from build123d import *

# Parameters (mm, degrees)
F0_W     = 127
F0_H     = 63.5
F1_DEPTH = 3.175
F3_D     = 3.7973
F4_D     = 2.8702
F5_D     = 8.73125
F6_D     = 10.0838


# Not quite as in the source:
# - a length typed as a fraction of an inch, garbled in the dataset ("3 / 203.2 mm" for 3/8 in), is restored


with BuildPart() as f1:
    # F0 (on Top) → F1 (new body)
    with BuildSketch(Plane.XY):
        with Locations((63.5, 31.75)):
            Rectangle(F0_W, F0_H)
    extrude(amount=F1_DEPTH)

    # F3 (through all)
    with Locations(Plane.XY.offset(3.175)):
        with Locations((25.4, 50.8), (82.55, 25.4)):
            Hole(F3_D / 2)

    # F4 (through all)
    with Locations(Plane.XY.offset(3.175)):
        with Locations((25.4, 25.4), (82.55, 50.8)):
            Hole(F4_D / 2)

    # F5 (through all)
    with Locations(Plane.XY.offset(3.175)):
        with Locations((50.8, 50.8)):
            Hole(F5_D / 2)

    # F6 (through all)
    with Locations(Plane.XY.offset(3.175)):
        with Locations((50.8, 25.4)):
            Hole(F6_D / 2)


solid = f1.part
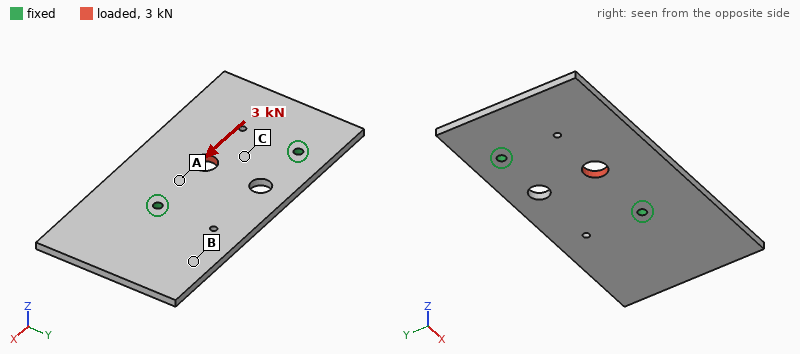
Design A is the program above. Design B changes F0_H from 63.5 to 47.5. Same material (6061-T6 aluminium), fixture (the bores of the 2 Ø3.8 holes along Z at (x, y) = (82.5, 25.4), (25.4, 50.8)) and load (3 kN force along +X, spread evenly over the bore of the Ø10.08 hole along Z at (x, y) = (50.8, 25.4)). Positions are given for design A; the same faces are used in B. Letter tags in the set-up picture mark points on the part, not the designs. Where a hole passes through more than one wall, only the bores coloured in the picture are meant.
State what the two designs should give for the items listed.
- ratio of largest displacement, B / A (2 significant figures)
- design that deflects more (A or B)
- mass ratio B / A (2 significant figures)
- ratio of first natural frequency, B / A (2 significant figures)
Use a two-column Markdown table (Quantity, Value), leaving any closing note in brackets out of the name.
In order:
| Quantity | Value |
|---|---|
| ratio of largest displacement, B / A | 1.4 |
| design that deflects more | B |
| mass ratio B / A | 0.74 |
| ratio of first natural frequency, B / A | 1.1 |
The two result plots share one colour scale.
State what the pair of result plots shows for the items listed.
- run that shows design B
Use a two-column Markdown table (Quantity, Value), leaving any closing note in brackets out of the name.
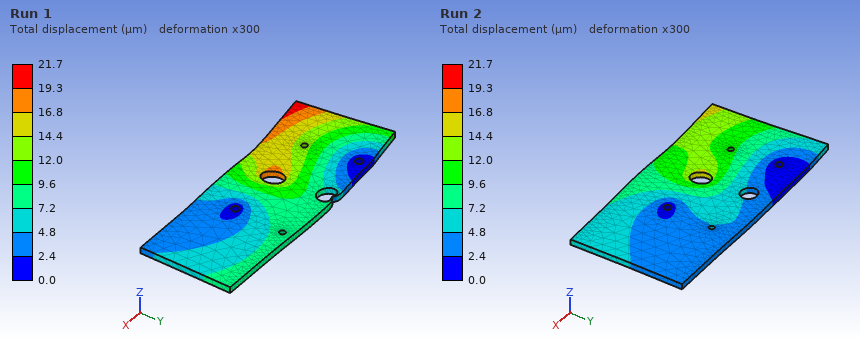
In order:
| Quantity | Value |
|---|---|
| run that shows design B | Run 1 |
